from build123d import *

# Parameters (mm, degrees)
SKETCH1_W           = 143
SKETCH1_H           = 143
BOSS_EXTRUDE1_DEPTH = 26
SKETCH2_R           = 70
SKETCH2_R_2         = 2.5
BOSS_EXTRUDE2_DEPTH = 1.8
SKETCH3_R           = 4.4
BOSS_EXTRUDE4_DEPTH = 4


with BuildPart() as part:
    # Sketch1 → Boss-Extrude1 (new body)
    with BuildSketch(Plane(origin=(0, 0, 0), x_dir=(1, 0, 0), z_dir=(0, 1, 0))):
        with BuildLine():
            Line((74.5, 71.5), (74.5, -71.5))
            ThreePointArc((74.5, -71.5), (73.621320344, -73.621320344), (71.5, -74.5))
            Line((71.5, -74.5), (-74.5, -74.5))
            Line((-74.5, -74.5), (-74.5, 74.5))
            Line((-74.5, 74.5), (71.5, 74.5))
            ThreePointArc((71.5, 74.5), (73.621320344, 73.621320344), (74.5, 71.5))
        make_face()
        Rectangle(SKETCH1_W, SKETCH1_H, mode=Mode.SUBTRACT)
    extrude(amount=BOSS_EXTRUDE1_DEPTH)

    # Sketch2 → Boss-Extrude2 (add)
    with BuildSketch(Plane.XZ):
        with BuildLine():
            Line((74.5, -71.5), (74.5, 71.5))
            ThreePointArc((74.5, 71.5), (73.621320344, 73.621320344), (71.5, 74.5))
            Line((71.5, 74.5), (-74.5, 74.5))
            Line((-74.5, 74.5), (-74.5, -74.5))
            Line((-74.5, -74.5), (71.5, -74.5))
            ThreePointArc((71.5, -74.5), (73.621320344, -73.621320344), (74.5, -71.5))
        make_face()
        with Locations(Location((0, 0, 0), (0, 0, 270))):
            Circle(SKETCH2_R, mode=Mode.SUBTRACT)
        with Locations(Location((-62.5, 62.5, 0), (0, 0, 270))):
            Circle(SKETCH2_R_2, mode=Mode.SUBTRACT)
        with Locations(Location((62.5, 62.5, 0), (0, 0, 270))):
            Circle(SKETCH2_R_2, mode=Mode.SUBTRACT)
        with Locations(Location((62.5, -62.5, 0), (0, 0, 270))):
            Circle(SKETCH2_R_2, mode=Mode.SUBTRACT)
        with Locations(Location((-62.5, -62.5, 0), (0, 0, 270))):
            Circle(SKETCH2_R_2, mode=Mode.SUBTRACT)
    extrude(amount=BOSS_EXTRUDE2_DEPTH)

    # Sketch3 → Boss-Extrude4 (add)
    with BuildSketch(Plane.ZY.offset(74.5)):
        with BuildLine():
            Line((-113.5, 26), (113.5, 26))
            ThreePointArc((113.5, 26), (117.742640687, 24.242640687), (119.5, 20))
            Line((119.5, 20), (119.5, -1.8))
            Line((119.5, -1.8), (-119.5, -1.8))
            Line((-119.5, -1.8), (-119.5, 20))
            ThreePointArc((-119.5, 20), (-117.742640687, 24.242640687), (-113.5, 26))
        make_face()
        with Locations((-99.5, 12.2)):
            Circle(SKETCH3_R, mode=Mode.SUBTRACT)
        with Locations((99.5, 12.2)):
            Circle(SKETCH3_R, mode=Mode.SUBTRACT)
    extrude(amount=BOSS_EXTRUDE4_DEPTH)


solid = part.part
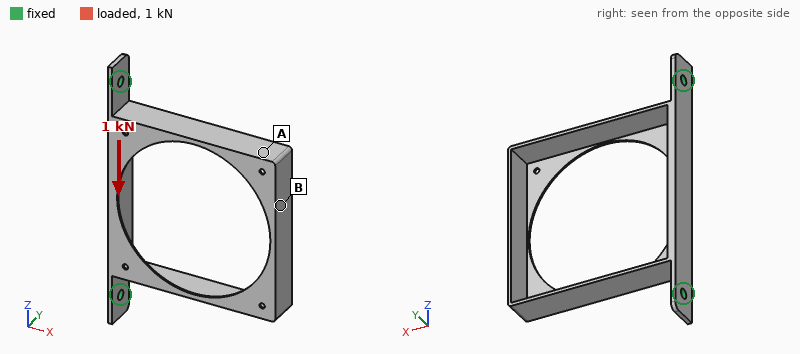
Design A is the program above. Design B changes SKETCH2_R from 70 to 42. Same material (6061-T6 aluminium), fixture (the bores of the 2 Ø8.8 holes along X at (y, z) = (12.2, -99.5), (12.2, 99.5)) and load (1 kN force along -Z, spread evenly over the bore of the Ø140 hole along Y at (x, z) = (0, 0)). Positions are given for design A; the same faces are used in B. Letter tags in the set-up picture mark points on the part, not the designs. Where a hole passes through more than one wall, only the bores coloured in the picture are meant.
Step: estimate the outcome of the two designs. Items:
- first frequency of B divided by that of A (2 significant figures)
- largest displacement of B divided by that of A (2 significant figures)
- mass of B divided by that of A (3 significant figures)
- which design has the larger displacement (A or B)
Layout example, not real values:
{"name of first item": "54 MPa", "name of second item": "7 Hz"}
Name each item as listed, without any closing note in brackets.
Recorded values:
{"first frequency of B divided by that of A": "0.90", "largest displacement of B divided by that of A": "0.37", "mass of B divided by that of A": "1.21", "which design has the larger displacement": "A"}
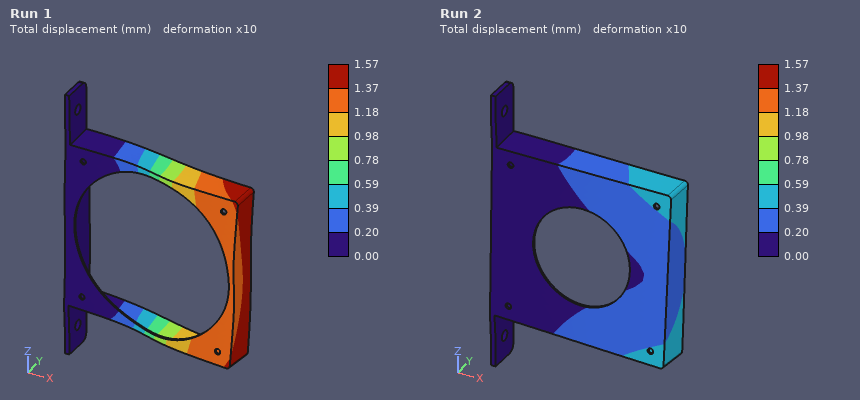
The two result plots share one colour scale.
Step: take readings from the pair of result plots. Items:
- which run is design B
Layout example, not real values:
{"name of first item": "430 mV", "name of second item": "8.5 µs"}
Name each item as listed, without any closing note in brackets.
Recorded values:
{"which run is design B": "Run 2"}
